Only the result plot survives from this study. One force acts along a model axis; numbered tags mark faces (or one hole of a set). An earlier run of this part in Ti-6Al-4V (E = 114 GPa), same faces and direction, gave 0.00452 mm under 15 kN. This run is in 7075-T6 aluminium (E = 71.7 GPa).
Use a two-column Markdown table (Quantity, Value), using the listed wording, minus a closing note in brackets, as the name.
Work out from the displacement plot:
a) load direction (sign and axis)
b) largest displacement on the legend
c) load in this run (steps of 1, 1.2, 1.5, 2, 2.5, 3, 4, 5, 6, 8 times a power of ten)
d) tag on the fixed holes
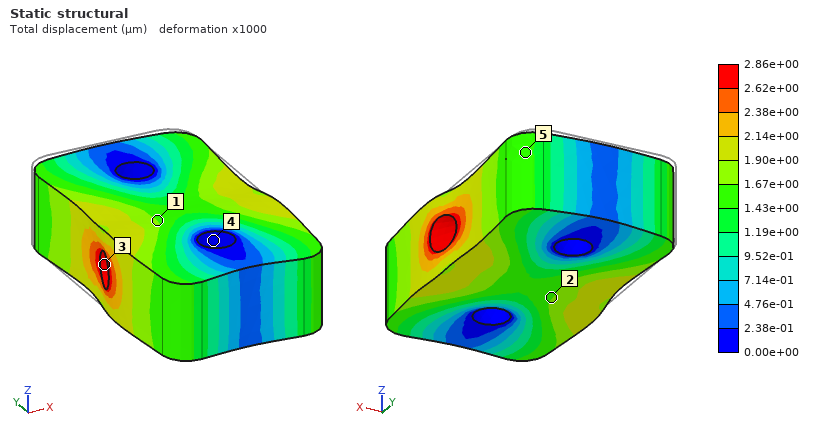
| Quantity | Value |
|---|---|
| load direction | -Y |
| largest displacement on the legend | 2.86e+00 µm |
| load in this run | 6 kN |
| tag on the fixed holes | 4 |
